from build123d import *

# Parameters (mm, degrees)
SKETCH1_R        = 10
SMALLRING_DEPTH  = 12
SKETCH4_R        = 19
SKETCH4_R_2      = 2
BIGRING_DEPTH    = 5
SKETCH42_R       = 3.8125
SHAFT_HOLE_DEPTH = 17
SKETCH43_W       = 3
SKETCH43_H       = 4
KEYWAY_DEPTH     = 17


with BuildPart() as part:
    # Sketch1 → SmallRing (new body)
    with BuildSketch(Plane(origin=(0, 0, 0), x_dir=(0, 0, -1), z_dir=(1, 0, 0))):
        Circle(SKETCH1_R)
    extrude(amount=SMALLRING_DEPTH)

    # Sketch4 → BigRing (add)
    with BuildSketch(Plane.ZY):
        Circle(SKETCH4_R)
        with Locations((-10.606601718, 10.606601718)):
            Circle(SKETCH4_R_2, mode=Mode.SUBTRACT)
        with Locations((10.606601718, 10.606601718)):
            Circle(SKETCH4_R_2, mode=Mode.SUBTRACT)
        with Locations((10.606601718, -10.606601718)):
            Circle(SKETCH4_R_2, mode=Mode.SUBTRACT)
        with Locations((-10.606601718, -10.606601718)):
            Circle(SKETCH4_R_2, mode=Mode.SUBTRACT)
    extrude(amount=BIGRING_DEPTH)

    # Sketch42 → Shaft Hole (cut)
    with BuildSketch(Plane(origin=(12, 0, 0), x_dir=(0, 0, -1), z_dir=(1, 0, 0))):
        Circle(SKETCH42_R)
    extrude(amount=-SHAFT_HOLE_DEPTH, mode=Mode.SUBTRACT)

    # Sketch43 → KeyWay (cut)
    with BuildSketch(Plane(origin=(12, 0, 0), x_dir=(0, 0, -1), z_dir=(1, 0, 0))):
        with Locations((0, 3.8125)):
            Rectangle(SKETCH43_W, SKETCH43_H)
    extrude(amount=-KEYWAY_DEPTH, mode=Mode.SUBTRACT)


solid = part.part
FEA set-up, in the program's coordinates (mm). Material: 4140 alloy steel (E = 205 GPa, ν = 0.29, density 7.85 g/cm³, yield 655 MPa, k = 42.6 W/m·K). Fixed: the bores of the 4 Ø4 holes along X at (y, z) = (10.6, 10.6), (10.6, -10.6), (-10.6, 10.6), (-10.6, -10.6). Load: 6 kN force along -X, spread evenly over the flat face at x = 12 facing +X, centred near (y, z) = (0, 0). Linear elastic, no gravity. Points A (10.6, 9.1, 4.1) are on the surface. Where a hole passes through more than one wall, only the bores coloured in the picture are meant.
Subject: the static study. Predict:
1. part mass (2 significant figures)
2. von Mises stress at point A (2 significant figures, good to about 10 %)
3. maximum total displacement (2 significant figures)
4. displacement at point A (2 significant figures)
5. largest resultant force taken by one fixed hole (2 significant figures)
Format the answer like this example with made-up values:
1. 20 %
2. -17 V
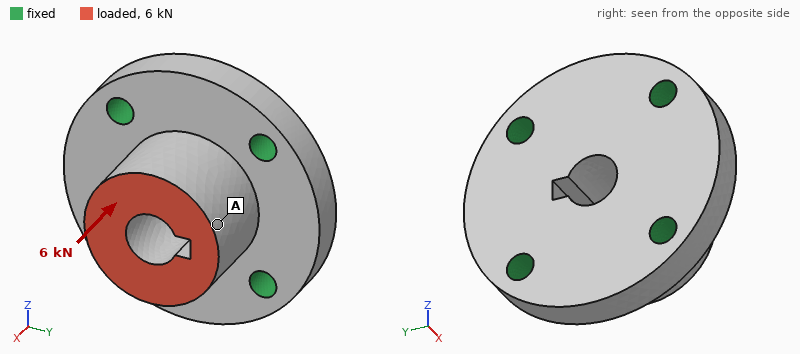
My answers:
1. 65 g
2. 22 MPa
3. 5.0 µm
4. 4.8 µm
5. 1.6 kN
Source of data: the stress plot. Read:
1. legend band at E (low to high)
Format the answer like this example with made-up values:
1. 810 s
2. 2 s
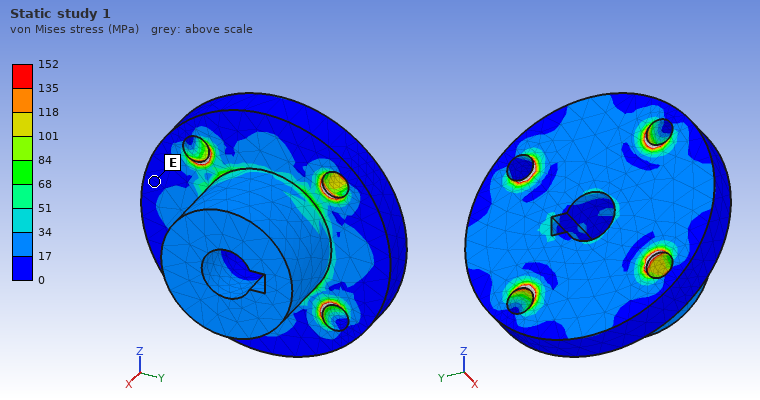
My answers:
1. 0 to 17 MPa
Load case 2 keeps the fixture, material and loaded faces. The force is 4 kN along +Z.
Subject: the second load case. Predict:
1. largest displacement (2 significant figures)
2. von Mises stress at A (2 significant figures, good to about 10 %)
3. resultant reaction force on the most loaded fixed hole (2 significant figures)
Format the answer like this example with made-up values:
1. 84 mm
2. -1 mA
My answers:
1. 14 µm
2. 27 MPa
3. 1.9 kN
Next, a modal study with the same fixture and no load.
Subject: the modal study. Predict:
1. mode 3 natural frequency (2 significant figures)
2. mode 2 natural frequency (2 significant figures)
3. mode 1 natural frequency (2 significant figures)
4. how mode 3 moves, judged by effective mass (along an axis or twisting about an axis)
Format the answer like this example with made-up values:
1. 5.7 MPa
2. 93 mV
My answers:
1. 31 kHz
2. 27 kHz
3. 27 kHz
4. along X
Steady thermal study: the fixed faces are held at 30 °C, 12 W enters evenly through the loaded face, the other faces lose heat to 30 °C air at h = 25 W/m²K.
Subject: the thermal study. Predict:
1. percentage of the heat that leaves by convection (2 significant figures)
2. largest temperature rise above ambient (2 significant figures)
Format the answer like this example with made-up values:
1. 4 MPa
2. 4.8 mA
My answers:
1. 4.7 %
2. 20 K
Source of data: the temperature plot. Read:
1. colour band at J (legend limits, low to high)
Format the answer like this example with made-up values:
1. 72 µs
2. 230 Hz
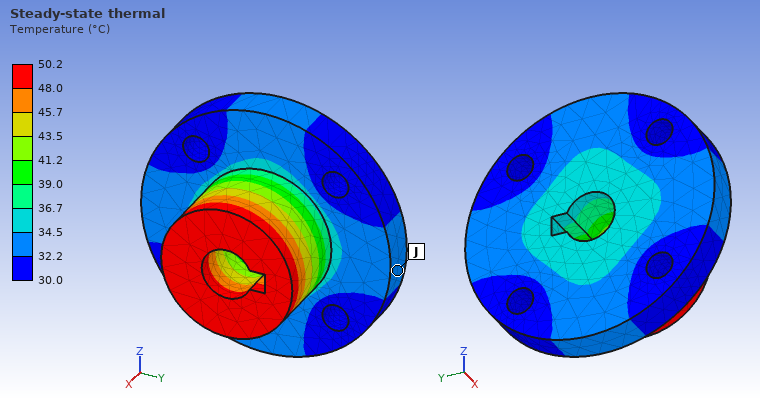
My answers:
1. 32.2 to 34.5 °C
